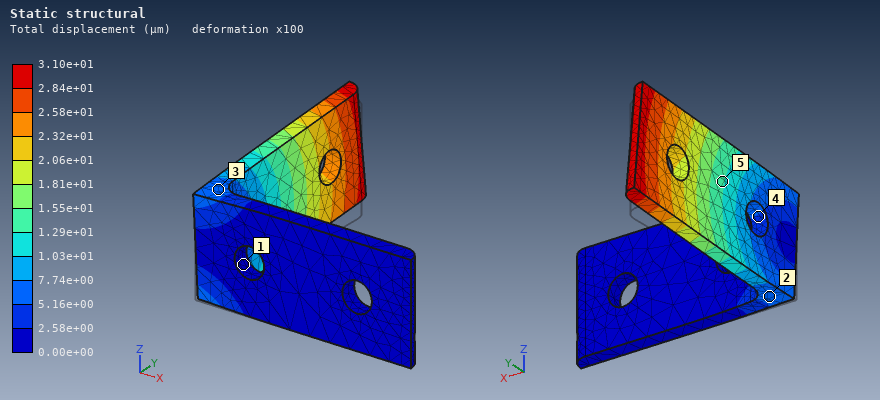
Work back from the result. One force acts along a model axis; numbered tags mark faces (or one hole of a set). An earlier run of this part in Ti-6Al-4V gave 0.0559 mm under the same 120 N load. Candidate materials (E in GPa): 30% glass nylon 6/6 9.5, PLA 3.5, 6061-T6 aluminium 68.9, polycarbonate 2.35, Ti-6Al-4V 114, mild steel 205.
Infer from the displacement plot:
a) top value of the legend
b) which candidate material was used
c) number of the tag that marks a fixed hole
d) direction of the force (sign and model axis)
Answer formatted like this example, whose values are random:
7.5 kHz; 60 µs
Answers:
3.10e+01 µm; mild steel; 1; +Z
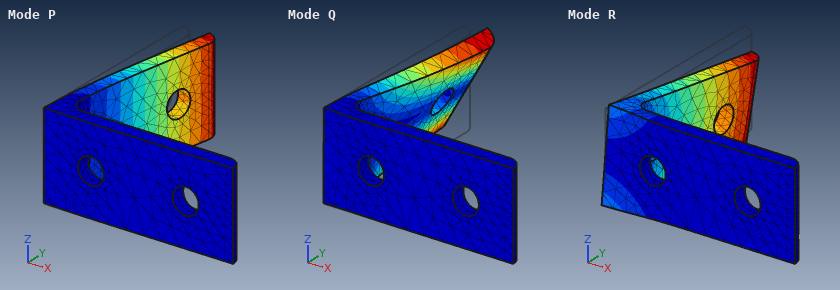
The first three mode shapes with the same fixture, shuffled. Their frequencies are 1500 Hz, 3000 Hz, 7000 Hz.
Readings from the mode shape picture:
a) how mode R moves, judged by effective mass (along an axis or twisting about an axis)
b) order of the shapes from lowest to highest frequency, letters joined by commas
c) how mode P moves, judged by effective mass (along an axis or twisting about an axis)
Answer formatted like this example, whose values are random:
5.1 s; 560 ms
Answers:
along Z; P, R, Q; along X
